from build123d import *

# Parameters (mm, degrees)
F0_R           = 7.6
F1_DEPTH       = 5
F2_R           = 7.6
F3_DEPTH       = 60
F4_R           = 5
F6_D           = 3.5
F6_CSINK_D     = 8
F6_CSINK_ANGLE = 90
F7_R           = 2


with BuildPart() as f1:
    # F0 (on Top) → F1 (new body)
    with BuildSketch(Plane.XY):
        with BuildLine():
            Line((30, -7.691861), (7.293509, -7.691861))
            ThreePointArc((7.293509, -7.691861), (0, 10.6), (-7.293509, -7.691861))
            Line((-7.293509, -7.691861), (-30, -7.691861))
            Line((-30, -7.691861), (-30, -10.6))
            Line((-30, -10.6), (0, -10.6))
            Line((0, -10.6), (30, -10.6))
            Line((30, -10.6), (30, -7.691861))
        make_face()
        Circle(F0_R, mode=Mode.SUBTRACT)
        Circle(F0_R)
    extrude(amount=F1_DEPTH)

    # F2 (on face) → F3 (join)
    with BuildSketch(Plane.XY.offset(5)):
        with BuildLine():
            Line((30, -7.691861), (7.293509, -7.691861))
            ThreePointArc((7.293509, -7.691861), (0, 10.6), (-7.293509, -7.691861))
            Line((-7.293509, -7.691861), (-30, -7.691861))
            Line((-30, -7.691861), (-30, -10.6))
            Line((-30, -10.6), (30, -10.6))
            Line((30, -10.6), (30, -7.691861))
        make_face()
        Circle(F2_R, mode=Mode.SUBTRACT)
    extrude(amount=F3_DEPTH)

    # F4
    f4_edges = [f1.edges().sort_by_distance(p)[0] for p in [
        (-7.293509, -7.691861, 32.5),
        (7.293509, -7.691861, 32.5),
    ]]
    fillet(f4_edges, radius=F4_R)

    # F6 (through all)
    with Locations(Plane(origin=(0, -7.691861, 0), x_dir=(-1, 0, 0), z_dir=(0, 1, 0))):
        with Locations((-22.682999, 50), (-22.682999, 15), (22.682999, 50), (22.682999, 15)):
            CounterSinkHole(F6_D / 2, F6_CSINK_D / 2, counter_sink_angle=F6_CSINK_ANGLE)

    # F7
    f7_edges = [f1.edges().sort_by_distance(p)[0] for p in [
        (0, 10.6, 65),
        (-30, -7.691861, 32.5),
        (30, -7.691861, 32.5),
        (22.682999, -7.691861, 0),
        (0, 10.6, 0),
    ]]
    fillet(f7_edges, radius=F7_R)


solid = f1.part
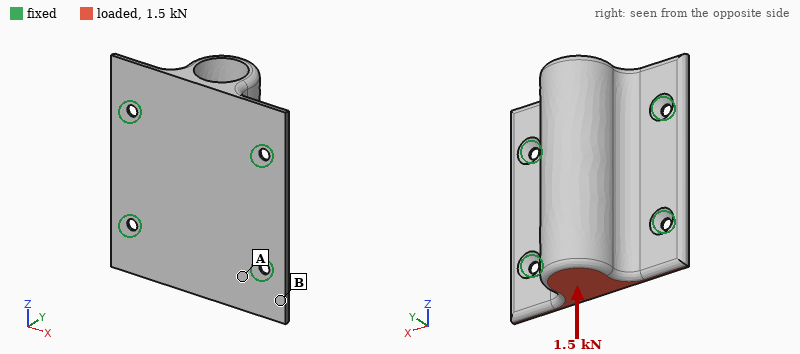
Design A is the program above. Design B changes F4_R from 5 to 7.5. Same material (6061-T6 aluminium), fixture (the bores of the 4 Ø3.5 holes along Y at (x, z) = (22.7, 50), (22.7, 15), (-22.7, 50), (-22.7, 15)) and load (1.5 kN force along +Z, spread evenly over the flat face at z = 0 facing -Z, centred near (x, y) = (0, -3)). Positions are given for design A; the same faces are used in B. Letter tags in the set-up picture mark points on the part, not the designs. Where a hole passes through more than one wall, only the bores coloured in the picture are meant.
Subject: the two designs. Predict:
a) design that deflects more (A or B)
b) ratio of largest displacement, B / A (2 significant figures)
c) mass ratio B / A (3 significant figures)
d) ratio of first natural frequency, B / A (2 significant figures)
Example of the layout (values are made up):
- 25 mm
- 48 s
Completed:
- A
- 0.74
- 1.05
- 1.1
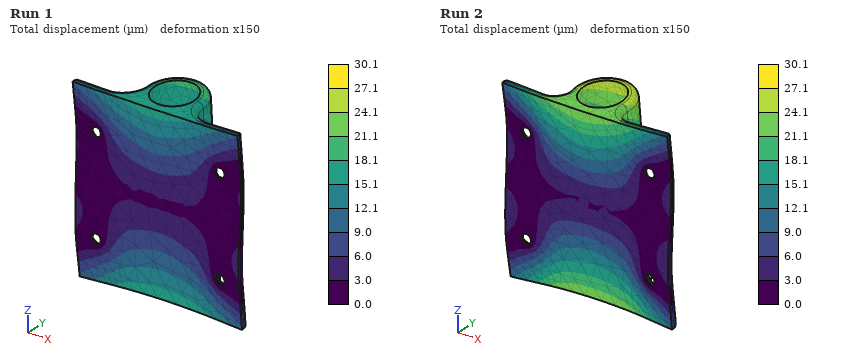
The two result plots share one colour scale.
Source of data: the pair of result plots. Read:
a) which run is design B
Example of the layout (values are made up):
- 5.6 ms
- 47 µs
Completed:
- Run 1
